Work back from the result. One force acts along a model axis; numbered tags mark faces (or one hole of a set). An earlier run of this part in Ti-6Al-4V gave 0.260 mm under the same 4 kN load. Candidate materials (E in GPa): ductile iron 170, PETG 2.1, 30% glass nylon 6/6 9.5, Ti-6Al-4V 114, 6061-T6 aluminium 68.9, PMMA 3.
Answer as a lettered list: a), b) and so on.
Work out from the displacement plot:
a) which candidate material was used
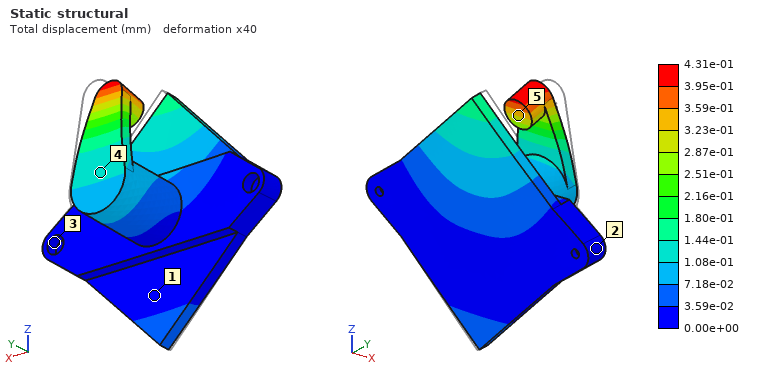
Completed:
a) 6061-T6 aluminium
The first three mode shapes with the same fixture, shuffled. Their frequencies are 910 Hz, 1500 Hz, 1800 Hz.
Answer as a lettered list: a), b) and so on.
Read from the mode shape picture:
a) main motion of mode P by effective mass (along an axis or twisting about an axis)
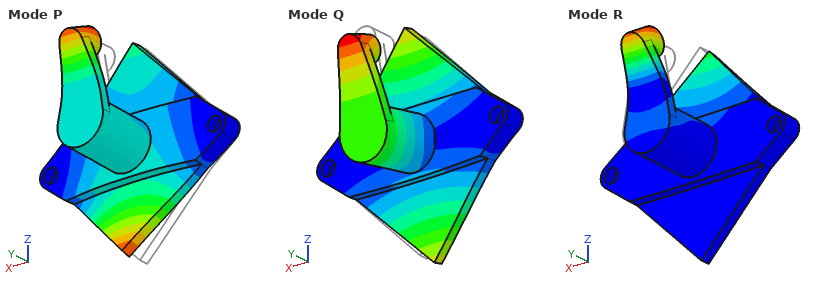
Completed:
a) along Y
